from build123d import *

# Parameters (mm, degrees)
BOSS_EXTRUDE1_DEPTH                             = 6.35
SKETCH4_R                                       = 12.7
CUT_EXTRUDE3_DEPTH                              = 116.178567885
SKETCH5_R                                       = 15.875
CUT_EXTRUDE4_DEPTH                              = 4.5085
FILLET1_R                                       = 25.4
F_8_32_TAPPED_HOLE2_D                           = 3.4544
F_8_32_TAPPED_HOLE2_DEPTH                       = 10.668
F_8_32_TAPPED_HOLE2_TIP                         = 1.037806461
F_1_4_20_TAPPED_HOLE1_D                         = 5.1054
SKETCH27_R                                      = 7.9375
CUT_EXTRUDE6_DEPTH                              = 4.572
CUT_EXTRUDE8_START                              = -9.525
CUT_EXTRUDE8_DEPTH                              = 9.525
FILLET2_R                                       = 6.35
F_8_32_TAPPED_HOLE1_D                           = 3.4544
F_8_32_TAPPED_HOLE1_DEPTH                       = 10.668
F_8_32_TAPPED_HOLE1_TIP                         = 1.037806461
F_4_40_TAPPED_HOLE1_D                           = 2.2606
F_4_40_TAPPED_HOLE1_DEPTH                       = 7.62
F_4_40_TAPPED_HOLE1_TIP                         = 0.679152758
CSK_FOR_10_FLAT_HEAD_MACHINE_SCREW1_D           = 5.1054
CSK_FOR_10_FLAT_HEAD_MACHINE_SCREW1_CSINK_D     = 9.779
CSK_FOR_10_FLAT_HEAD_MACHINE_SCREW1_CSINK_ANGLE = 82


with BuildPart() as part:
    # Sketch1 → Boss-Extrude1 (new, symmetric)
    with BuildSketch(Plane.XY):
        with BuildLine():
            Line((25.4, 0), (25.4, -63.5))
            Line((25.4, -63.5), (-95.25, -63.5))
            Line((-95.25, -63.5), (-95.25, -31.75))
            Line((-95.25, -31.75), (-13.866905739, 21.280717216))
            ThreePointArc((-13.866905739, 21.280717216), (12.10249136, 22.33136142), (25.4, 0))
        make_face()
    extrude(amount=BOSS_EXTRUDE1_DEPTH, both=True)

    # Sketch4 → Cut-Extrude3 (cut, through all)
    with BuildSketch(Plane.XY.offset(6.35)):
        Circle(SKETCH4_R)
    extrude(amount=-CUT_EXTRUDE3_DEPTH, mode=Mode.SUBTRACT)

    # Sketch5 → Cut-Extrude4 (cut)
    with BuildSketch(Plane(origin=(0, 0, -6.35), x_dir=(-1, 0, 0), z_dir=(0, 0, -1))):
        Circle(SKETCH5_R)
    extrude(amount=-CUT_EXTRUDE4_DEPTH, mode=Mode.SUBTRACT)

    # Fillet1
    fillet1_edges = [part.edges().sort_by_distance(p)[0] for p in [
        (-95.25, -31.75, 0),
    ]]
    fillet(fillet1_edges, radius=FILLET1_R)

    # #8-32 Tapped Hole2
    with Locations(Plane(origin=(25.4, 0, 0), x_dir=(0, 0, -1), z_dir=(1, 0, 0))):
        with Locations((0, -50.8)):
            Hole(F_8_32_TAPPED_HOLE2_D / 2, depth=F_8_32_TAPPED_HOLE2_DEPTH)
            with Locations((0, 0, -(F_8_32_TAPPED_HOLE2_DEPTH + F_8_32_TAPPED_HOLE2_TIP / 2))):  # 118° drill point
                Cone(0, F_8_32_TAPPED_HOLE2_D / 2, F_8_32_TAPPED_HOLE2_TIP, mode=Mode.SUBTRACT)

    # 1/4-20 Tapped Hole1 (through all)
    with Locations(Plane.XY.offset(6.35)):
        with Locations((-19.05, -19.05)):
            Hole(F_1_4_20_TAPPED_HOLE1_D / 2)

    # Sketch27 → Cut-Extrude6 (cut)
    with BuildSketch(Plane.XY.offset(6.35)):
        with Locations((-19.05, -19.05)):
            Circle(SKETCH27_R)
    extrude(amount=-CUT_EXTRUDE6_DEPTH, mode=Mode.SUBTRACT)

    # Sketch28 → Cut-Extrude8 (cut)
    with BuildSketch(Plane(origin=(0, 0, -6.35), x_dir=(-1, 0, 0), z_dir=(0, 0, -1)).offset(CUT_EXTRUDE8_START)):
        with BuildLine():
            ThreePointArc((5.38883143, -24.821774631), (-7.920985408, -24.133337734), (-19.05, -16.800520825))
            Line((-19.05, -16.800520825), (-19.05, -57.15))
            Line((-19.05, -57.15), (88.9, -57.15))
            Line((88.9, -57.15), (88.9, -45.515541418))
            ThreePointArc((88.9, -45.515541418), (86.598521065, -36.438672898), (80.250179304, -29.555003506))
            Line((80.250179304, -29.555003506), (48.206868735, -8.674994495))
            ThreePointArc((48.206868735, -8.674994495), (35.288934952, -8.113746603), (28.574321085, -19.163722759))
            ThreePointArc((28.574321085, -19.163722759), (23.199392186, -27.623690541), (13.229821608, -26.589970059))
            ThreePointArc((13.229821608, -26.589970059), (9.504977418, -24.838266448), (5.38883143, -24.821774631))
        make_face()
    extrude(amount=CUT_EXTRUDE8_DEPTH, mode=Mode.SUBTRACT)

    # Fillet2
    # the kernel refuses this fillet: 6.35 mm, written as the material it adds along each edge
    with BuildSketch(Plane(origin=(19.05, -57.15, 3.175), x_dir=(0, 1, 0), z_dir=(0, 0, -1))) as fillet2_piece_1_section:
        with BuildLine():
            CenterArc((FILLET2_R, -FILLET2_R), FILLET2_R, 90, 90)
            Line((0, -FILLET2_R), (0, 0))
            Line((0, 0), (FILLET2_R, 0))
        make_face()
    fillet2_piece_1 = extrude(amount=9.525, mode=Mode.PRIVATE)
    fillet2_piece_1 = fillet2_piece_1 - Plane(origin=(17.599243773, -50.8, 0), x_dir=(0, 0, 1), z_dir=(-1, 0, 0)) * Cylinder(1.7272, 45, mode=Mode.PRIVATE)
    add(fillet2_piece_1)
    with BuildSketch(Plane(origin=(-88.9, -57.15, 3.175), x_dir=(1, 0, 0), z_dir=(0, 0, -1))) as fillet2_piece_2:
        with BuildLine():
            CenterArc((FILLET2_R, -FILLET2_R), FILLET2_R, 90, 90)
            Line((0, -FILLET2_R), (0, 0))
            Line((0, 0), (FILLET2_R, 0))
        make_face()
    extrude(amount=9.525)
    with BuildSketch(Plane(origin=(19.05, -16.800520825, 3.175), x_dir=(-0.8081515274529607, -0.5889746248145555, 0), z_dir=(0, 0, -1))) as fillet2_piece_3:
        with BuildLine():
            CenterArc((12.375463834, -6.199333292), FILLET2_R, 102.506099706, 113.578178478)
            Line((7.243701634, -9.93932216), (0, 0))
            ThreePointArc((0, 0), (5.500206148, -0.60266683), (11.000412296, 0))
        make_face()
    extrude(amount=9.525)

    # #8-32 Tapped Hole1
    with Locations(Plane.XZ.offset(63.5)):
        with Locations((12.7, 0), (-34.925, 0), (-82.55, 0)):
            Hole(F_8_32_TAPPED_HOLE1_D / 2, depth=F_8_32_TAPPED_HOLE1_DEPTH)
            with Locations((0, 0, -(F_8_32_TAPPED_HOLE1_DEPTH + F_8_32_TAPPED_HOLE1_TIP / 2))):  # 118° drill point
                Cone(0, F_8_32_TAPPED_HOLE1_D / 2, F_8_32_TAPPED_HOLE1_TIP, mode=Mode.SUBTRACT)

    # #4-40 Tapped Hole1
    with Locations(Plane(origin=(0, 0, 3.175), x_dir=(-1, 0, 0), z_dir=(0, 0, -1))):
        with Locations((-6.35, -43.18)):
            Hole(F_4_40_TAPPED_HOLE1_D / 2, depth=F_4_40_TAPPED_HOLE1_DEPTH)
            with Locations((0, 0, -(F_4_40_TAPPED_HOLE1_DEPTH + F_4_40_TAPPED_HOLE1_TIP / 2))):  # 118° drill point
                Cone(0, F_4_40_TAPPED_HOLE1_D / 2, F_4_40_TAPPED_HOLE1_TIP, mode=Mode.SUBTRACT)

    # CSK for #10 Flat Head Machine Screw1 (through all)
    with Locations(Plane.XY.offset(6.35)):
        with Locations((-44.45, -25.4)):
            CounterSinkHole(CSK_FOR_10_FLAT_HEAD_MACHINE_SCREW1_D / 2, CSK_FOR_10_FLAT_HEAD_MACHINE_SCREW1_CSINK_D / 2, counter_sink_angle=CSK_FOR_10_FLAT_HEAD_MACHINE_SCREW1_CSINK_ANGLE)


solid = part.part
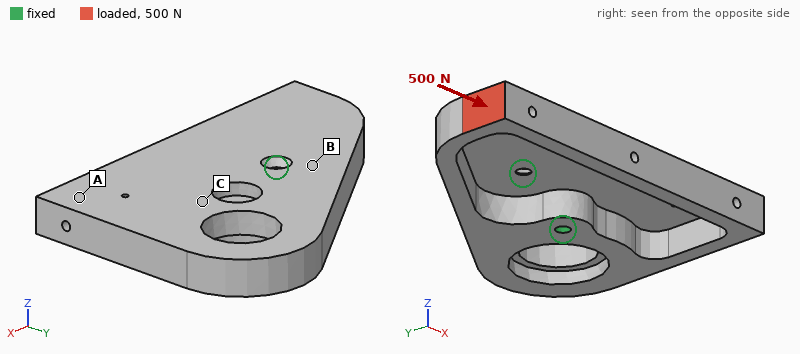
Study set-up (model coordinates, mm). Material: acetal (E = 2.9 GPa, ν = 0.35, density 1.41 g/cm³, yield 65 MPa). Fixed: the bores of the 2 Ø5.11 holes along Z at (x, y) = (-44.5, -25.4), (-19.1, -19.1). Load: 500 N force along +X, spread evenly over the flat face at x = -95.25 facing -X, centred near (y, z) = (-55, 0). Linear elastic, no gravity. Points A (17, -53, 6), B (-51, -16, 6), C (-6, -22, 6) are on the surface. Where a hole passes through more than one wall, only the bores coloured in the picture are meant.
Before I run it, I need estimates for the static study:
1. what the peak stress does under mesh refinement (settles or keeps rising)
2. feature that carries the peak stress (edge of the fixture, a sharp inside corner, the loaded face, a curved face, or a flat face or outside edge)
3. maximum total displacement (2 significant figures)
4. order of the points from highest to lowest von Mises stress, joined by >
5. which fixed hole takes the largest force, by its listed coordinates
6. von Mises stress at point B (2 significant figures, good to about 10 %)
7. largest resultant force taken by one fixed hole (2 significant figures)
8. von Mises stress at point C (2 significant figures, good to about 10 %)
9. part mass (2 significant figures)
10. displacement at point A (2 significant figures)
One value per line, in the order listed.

keeps rising
edge of the fixture
0.85 mm
B > C > A
(-44.5, -25.4)
6.4 MPa
590 N
4.2 MPa
79 g
0.48 mm
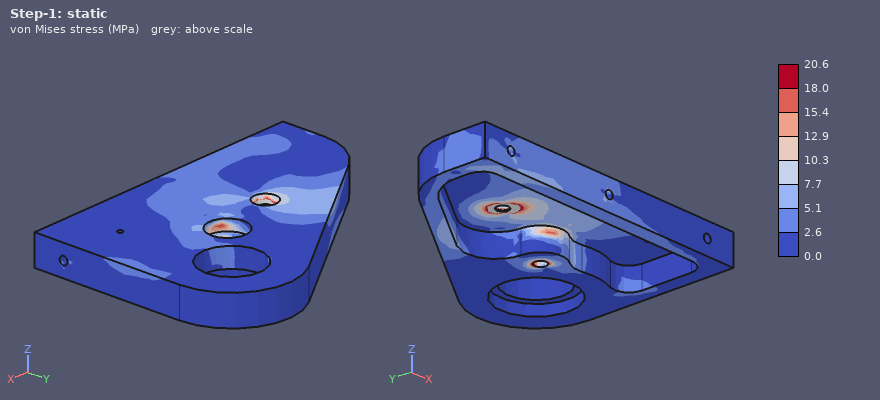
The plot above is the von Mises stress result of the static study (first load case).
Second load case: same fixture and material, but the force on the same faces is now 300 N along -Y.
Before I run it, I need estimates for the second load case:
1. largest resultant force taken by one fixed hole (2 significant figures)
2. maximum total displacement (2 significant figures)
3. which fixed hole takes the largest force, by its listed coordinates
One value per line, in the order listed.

710 N
0.83 mm
(-44.5, -25.4)
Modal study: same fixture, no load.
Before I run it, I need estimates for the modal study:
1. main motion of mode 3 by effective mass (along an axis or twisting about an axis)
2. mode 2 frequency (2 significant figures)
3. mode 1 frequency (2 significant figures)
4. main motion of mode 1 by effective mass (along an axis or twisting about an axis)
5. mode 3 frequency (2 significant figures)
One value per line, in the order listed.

along Z
430 Hz
300 Hz
along Z
700 Hz
